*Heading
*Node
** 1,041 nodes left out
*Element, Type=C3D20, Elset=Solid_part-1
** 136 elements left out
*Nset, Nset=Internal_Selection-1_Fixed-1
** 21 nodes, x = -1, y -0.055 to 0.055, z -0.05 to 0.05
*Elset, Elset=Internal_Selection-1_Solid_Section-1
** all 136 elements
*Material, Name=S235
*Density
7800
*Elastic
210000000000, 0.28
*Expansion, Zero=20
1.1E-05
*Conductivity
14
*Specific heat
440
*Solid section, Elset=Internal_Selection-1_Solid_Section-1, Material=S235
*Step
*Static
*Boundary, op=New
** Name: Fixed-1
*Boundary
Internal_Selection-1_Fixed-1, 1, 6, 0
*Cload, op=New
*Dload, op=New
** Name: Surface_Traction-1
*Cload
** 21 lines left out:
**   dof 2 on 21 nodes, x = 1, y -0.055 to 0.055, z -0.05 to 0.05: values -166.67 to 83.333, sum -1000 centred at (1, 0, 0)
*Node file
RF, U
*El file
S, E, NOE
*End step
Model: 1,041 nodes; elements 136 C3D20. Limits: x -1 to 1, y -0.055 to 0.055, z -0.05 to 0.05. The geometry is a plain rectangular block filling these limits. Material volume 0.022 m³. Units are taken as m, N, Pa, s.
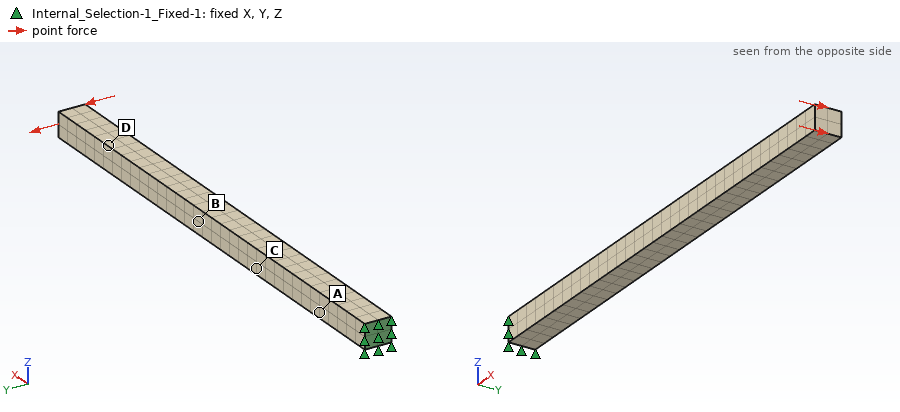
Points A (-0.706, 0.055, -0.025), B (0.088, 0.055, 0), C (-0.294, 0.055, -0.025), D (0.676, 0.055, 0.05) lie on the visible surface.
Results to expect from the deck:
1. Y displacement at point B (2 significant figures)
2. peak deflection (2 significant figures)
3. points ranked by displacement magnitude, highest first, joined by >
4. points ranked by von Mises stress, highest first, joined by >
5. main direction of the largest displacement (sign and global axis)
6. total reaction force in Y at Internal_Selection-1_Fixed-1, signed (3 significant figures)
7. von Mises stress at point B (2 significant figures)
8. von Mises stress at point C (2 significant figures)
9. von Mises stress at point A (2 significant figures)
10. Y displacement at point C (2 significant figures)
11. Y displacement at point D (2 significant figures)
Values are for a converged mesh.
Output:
-4.2e-04 m
0.0011 m
D > B > C > A
A > C > B > D
-Y
1000 N
4.5e+06 Pa
6.4e+06 Pa
8.5e+06 Pa
-1.9e-04 m
-8.7e-04 m
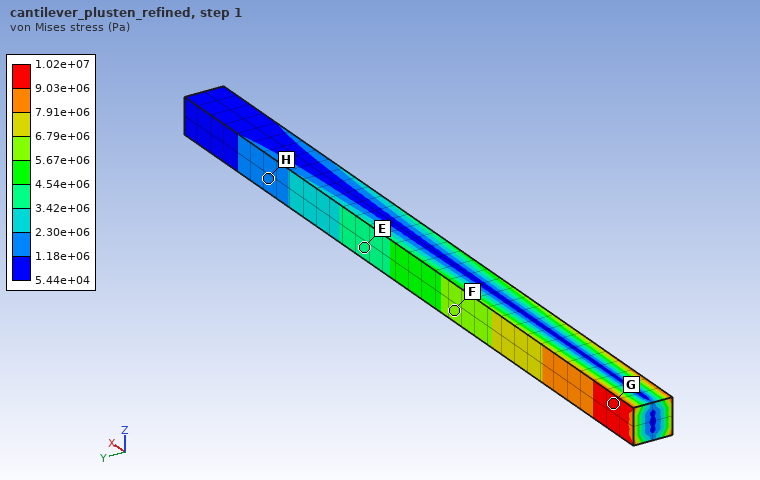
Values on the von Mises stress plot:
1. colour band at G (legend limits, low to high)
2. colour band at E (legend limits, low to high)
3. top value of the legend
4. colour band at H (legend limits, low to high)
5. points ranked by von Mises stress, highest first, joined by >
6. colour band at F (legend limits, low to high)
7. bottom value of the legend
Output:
9.03e+06 to 1.02e+07 Pa
3.42e+06 to 4.54e+06 Pa
1.02e+07 Pa
1.18e+06 to 2.30e+06 Pa
G > F > E > H
5.67e+06 to 6.79e+06 Pa
5.44e+04 Pa
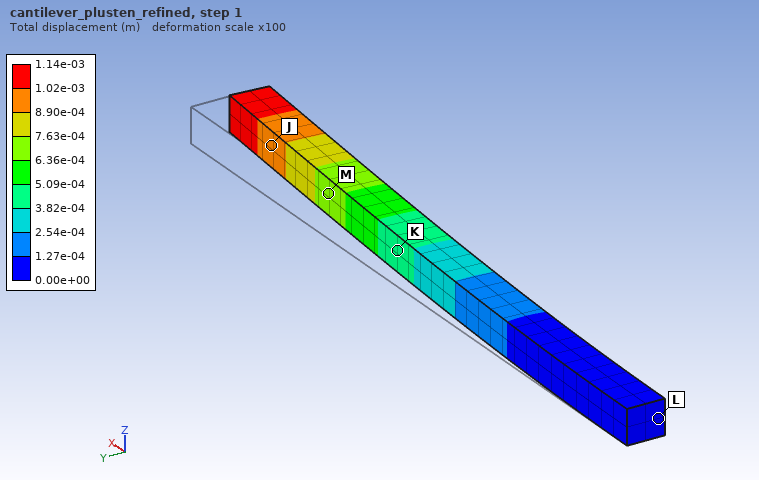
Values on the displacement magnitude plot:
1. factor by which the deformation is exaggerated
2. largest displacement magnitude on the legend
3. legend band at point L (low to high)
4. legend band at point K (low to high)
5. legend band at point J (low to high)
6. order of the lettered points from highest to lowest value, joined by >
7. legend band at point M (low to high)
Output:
100
1.14e-03 m
0.00e+00 to 1.27e-04 m
3.82e-04 to 5.09e-04 m
8.90e-04 to 1.02e-03 m
J > M > K > L
6.36e-04 to 7.63e-04 m
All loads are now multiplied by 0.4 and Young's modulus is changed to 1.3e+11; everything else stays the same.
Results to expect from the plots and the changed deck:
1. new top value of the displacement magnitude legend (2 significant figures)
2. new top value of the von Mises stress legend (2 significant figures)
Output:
7.4e-04 m
4.1e+06 Pa
